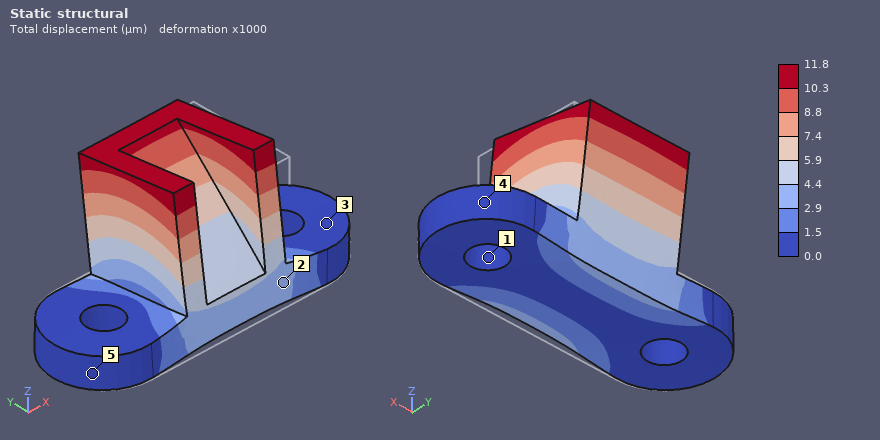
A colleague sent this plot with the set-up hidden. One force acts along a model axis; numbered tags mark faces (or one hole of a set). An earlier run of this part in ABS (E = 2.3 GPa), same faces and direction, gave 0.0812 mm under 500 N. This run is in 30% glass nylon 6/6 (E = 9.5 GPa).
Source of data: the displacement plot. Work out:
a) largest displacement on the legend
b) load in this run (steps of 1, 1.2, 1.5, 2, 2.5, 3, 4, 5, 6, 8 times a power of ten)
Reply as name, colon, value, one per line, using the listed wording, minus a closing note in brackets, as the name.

largest displacement on the legend: 11.8 µm
load in this run: 300 N
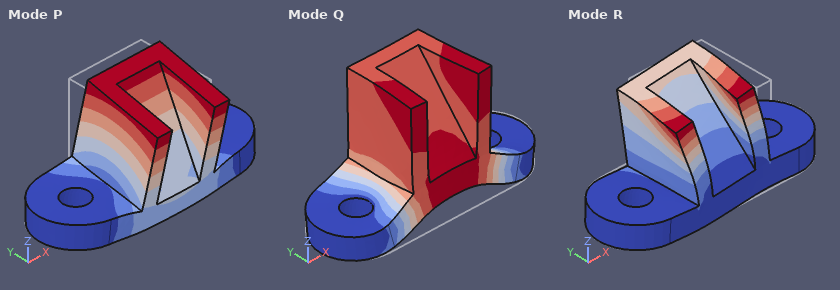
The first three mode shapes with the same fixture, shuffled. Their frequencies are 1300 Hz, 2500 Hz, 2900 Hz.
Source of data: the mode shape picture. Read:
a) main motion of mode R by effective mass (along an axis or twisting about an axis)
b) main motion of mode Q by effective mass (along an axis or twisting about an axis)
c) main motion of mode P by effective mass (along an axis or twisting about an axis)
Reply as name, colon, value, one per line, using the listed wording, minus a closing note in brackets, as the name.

main motion of mode R by effective mass: along X
main motion of mode Q by effective mass: along Z
main motion of mode P by effective mass: along Y
